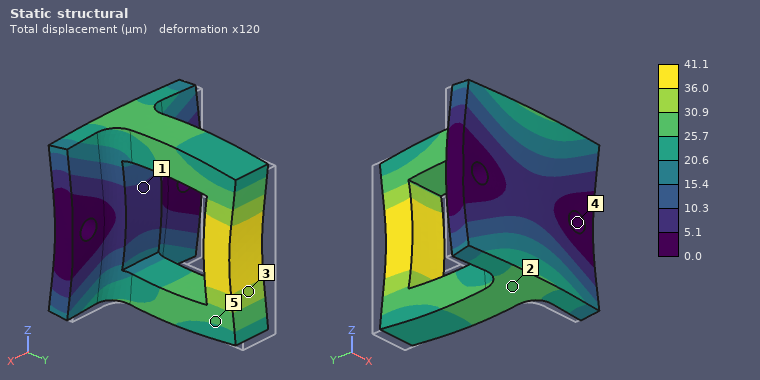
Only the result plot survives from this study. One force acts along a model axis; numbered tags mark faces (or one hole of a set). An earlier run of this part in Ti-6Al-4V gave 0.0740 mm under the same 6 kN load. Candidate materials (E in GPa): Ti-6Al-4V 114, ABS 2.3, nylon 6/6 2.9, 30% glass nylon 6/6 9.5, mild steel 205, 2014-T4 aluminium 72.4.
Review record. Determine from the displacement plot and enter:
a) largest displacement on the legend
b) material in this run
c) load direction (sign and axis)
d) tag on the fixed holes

41.1 µm
mild steel
-Y
4
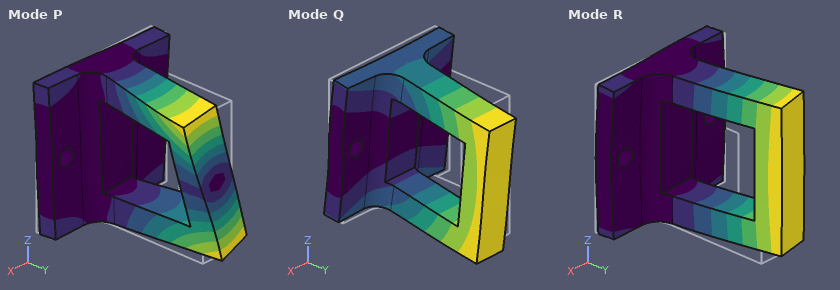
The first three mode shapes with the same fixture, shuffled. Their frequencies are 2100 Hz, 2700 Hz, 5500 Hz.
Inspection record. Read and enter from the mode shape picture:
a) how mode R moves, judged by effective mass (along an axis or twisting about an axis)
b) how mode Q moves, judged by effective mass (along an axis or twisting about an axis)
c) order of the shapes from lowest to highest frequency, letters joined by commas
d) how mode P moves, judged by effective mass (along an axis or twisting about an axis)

along X
along Z
Q, R, P
twisting about Y
